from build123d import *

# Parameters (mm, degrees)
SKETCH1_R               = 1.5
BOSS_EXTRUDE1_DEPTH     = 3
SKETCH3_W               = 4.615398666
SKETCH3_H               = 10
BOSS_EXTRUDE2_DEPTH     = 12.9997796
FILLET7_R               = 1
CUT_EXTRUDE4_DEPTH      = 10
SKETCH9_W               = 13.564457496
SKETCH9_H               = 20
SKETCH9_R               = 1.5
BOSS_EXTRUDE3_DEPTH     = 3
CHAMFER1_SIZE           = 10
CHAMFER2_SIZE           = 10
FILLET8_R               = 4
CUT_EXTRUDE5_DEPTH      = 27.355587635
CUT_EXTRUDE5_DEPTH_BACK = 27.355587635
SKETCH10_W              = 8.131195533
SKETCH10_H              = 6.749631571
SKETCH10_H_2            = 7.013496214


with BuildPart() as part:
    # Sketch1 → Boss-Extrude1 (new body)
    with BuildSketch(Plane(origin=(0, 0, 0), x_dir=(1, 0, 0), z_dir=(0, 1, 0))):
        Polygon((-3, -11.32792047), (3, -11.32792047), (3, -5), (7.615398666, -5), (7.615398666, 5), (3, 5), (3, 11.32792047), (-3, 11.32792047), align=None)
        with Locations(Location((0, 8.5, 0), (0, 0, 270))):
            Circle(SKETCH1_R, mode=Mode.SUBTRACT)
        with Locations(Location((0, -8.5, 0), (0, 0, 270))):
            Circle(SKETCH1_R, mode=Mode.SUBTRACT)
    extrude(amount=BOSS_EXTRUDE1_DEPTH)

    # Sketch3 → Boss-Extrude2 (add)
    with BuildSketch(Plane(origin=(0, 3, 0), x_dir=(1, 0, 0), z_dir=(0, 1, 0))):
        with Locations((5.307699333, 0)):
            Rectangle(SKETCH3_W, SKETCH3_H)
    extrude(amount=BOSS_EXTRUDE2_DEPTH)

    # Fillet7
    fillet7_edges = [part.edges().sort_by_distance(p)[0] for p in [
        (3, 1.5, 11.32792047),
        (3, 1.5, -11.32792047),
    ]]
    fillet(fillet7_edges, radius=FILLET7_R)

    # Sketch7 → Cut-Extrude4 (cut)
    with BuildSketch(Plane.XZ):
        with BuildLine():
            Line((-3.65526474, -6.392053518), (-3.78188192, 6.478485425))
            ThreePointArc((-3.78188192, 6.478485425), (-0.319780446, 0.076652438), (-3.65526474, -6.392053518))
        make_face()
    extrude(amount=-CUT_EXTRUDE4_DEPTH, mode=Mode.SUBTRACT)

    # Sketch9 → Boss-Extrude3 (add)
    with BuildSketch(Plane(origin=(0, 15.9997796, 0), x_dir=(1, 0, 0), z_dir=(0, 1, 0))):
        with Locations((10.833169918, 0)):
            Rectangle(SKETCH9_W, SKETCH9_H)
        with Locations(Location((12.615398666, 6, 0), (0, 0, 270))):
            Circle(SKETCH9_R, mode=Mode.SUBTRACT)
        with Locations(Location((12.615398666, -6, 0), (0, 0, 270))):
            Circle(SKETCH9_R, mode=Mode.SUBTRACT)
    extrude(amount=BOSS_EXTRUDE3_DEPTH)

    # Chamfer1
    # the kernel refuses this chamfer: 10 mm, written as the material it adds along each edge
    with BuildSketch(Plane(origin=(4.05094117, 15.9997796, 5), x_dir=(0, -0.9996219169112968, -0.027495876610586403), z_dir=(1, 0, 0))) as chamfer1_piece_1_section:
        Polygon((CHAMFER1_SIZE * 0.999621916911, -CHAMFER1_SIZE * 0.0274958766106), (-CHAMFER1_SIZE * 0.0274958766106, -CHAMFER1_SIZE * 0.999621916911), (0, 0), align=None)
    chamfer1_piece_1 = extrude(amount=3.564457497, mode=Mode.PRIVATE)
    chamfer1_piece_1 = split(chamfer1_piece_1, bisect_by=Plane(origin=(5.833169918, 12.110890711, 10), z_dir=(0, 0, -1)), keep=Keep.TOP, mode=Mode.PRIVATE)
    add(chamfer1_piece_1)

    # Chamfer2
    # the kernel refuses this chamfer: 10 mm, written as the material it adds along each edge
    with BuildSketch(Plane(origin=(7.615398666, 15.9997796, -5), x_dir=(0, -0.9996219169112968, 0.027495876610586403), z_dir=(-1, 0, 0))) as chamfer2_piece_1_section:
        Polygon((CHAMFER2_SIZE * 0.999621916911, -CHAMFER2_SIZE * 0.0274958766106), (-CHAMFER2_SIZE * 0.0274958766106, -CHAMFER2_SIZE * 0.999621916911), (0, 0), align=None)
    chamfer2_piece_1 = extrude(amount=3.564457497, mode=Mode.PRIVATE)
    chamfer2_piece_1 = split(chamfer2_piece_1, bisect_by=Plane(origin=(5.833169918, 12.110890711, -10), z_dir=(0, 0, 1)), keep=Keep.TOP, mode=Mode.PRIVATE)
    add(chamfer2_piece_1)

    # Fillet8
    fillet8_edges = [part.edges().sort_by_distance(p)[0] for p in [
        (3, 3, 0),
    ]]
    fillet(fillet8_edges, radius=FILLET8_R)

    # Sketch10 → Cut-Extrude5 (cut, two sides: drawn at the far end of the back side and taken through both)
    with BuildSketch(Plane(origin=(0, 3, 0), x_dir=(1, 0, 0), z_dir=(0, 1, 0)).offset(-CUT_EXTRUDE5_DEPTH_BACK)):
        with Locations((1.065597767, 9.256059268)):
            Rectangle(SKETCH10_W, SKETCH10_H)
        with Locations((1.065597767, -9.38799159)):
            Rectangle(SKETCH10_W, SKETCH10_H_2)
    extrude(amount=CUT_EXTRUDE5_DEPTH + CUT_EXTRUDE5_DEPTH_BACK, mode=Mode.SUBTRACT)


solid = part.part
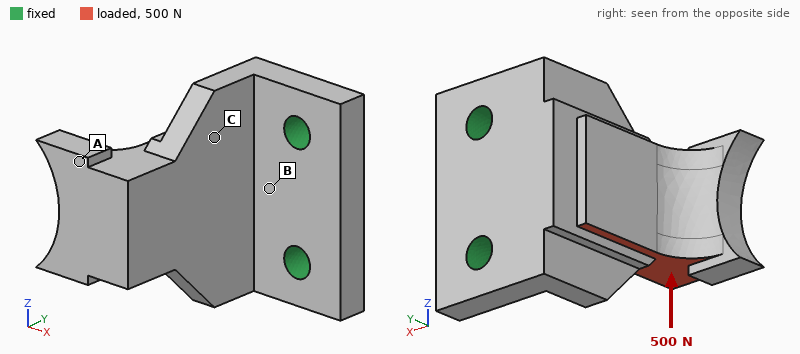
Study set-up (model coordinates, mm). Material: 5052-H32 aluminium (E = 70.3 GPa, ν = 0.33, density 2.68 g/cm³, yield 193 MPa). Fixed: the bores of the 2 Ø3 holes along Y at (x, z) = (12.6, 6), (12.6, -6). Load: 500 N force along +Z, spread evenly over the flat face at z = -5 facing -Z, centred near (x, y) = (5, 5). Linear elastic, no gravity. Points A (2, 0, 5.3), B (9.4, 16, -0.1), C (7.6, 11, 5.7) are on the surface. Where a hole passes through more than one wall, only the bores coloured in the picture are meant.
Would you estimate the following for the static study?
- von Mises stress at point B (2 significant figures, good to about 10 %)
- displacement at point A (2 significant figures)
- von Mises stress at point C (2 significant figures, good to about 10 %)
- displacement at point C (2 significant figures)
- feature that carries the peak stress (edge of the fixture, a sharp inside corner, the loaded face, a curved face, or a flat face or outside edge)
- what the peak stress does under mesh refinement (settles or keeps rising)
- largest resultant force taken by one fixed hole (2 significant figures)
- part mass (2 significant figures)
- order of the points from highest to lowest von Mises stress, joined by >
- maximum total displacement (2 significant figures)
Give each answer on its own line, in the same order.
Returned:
56 MPa
43 µm
30 MPa
21 µm
edge of the fixture
keeps rising
580 N
5.0 g
B > C > A
47 µm
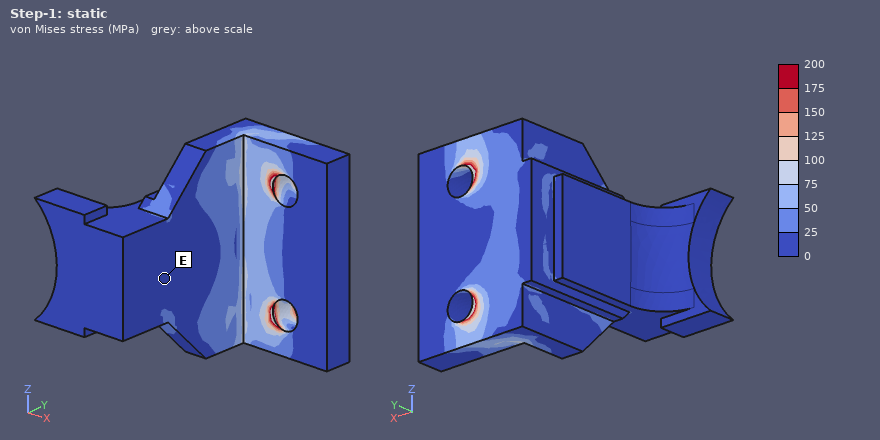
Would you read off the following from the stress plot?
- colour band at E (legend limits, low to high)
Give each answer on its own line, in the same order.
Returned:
0 to 25 MPa
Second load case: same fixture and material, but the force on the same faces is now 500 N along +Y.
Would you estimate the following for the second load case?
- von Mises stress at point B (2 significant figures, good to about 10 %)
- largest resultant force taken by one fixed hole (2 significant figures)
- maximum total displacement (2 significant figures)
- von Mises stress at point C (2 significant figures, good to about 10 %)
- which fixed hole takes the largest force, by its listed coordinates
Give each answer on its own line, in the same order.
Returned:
58 MPa
430 N
0.12 mm
17 MPa
(12.6, -6)
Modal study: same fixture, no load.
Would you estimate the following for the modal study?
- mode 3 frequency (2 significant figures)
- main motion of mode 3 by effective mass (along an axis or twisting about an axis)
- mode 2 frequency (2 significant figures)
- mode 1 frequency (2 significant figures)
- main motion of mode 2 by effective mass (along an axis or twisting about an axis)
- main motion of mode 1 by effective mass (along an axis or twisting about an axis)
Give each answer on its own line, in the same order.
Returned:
22 kHz
along Y
13 kHz
4900 Hz
along Z
along X
